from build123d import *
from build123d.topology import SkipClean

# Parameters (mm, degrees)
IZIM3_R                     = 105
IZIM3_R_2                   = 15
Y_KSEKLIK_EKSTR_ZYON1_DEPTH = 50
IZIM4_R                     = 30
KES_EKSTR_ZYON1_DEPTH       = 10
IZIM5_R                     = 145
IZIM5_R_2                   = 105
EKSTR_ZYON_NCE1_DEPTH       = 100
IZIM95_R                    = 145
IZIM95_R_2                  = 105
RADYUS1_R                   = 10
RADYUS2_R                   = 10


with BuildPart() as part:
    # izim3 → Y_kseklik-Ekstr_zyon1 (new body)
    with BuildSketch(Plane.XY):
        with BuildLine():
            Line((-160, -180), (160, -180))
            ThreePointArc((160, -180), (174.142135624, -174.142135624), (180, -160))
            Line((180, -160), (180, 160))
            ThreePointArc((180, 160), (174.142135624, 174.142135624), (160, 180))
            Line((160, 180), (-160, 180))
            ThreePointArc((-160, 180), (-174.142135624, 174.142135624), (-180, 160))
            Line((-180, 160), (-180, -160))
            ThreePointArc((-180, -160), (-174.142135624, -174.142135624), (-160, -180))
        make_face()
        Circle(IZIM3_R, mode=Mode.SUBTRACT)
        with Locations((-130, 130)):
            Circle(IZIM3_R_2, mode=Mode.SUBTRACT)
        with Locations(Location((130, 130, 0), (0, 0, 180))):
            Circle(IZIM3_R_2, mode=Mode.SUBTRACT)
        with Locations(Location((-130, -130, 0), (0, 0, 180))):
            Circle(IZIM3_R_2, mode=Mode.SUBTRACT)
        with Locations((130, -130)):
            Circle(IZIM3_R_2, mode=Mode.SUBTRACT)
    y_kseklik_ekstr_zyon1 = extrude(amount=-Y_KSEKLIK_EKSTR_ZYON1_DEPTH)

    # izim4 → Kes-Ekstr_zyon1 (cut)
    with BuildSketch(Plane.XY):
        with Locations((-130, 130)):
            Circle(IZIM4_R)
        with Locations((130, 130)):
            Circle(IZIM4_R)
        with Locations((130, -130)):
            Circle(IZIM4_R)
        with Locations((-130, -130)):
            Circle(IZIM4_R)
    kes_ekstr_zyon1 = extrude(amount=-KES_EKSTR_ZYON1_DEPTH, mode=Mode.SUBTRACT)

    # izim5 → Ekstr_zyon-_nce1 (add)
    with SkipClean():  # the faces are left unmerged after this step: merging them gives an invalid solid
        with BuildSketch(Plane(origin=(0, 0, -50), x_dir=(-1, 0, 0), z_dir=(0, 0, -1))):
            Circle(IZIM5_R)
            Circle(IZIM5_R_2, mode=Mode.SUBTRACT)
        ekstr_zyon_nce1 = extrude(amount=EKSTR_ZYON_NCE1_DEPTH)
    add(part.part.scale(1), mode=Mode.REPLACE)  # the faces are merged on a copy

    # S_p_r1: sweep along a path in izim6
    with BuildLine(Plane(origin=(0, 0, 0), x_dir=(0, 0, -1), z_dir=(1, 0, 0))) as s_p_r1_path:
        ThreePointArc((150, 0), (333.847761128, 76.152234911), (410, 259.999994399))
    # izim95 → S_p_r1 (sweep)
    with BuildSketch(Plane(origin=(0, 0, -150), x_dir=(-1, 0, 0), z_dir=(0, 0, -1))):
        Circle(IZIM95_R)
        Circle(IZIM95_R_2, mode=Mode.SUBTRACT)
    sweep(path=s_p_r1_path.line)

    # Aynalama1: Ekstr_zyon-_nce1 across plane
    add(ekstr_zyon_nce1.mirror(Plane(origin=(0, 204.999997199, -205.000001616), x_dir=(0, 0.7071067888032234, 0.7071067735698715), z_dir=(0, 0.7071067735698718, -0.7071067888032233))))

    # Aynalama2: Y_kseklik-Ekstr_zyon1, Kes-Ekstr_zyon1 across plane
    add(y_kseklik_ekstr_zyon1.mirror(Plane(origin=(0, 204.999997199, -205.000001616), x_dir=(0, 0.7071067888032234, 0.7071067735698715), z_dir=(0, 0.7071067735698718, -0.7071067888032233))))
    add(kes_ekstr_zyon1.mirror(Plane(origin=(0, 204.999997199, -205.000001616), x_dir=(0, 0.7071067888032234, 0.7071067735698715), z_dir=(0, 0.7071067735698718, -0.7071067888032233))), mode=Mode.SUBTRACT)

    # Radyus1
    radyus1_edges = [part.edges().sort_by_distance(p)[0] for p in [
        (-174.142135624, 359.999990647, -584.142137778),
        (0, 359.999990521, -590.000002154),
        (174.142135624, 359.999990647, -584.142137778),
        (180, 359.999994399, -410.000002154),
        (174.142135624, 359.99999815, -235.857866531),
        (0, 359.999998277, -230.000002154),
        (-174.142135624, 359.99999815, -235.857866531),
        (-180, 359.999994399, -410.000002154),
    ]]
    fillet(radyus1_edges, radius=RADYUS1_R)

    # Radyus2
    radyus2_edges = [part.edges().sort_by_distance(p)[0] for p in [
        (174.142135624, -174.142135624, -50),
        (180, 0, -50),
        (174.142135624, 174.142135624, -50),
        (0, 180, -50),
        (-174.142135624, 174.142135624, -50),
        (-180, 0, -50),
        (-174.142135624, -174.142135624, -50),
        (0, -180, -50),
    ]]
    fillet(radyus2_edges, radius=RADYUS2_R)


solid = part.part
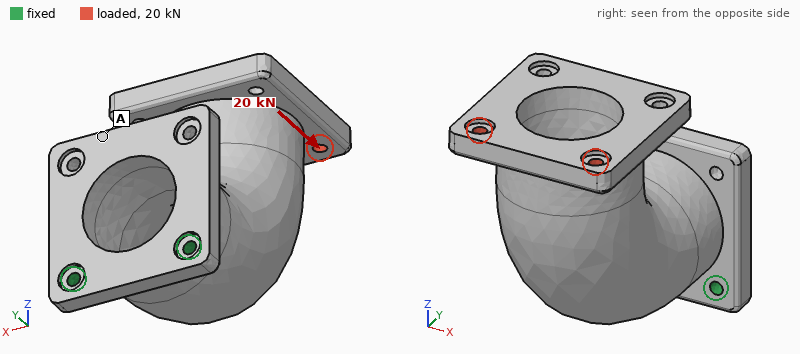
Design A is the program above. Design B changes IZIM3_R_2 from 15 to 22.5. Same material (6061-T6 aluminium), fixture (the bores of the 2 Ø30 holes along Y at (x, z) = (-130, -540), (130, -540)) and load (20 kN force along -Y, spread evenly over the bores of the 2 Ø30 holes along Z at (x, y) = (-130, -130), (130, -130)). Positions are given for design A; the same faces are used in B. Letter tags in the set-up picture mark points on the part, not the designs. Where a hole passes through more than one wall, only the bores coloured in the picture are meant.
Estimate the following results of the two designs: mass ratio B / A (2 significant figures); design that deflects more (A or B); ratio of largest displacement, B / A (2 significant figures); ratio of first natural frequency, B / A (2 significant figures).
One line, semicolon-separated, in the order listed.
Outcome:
0.99; A; 0.75; 1.2
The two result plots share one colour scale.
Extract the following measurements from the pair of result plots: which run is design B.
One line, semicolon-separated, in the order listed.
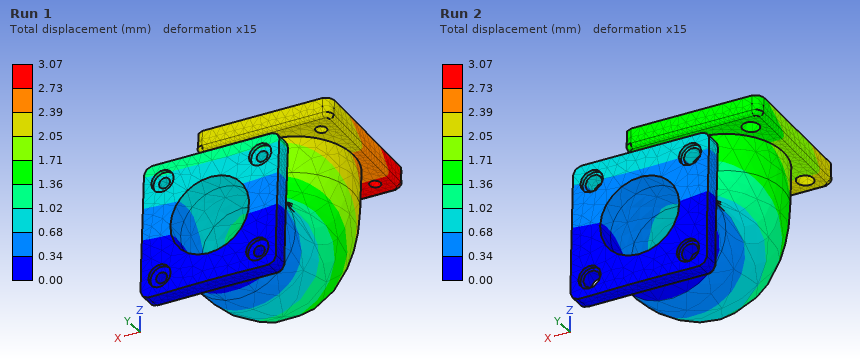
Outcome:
Run 2
